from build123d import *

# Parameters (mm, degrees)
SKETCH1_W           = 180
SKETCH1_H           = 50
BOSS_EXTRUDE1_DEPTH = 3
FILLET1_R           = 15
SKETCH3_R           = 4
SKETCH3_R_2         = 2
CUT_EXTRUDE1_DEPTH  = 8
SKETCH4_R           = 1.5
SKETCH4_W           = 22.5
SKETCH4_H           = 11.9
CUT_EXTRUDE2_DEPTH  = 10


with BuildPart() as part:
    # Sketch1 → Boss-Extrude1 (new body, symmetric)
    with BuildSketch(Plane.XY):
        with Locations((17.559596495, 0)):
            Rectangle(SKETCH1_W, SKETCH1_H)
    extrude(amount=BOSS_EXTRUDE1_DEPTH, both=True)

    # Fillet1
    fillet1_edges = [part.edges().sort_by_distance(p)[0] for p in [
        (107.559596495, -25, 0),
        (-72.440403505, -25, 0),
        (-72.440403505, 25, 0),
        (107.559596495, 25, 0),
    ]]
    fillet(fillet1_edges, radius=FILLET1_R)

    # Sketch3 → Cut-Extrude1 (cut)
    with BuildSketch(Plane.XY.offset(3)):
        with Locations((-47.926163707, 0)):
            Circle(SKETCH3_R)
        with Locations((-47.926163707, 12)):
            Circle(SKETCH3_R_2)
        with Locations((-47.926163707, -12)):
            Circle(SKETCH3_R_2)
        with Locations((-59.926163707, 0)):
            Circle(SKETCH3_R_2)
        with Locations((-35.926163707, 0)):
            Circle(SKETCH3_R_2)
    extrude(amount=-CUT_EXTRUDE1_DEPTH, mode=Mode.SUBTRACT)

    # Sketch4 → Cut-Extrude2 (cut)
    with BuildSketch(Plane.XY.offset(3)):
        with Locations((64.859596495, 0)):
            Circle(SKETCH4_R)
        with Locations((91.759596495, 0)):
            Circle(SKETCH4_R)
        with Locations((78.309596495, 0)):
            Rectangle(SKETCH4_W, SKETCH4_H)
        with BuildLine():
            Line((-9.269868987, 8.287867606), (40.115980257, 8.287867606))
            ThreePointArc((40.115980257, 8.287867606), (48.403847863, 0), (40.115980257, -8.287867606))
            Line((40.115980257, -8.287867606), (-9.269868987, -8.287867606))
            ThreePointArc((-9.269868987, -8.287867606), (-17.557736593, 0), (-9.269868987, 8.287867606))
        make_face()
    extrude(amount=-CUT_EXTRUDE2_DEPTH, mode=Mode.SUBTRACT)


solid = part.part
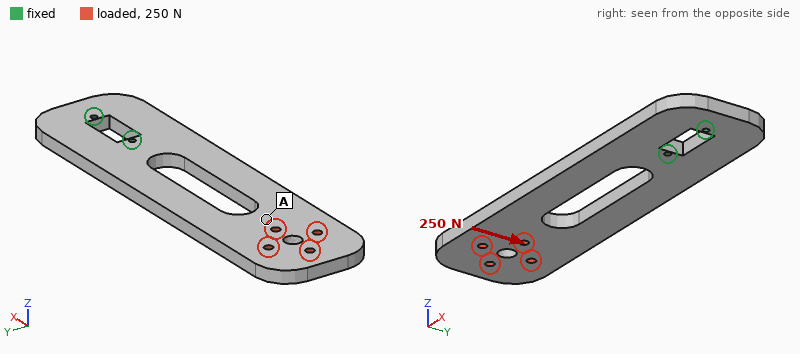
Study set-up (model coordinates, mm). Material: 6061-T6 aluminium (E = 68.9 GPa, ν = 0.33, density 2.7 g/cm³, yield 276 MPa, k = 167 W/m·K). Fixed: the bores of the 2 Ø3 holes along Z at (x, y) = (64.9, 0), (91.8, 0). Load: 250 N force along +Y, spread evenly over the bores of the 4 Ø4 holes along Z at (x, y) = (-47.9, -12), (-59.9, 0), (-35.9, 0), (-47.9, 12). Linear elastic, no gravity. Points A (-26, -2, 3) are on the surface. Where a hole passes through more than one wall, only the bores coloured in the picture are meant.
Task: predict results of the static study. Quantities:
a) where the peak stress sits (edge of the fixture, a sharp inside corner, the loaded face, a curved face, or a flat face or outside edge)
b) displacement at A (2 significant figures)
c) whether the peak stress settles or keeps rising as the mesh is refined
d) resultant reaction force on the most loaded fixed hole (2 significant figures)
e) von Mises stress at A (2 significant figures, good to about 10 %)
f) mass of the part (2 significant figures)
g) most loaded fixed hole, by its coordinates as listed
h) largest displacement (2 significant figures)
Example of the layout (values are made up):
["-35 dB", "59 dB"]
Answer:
["edge of the fixture", "0.097 mm", "keeps rising", "1.1 kN", "6.0 MPa", "120 g", "(64.9, 0)", "0.14 mm"]
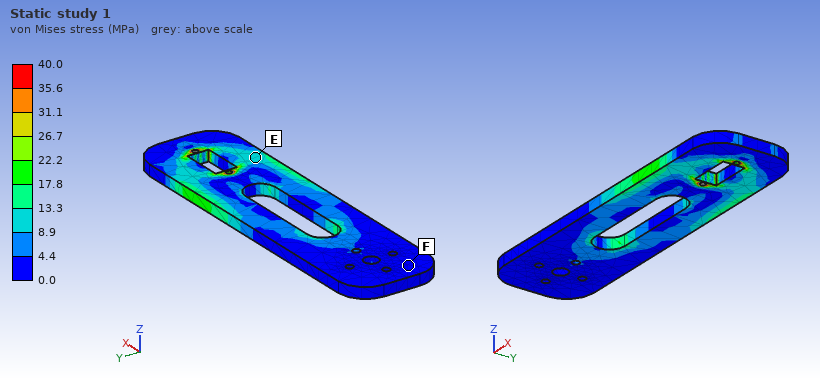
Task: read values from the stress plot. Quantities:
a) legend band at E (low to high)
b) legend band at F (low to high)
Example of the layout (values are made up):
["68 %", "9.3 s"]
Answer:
["8.9 to 13.3 MPa", "0.0 to 4.4 MPa"]
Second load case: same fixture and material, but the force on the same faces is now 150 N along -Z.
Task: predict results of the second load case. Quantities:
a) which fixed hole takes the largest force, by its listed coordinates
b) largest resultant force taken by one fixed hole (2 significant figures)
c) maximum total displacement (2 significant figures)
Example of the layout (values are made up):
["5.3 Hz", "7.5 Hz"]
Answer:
["(64.9, 0)", "490 N", "2.2 mm"]
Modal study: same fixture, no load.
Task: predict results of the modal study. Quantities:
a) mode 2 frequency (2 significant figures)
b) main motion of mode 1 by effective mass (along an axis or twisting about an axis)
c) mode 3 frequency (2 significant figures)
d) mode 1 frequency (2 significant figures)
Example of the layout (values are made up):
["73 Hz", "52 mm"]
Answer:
["1100 Hz", "along Z", "1100 Hz", "230 Hz"]
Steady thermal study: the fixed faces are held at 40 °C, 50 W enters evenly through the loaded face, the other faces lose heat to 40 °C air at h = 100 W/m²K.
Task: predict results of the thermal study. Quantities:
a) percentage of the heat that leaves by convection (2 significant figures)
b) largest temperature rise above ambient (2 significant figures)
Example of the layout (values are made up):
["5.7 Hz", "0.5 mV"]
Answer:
["82 %", "54 K"]
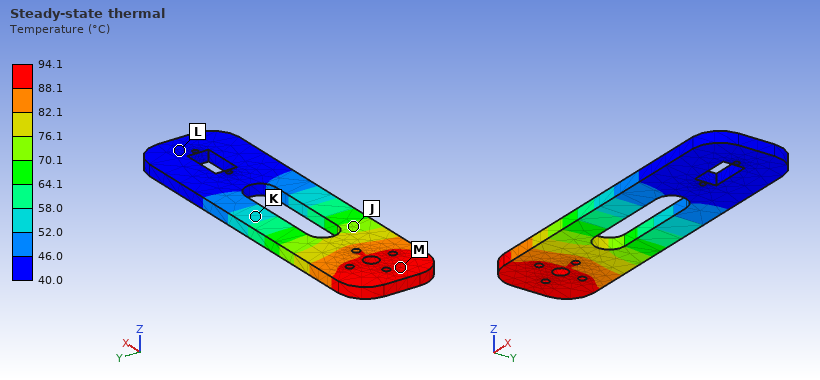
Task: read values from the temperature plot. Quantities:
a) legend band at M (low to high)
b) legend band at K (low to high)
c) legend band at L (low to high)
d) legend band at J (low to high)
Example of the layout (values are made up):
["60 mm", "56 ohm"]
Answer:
["88.1 to 94.1 °C", "52.0 to 58.0 °C", "40.0 to 46.0 °C", "70.1 to 76.1 °C"]
